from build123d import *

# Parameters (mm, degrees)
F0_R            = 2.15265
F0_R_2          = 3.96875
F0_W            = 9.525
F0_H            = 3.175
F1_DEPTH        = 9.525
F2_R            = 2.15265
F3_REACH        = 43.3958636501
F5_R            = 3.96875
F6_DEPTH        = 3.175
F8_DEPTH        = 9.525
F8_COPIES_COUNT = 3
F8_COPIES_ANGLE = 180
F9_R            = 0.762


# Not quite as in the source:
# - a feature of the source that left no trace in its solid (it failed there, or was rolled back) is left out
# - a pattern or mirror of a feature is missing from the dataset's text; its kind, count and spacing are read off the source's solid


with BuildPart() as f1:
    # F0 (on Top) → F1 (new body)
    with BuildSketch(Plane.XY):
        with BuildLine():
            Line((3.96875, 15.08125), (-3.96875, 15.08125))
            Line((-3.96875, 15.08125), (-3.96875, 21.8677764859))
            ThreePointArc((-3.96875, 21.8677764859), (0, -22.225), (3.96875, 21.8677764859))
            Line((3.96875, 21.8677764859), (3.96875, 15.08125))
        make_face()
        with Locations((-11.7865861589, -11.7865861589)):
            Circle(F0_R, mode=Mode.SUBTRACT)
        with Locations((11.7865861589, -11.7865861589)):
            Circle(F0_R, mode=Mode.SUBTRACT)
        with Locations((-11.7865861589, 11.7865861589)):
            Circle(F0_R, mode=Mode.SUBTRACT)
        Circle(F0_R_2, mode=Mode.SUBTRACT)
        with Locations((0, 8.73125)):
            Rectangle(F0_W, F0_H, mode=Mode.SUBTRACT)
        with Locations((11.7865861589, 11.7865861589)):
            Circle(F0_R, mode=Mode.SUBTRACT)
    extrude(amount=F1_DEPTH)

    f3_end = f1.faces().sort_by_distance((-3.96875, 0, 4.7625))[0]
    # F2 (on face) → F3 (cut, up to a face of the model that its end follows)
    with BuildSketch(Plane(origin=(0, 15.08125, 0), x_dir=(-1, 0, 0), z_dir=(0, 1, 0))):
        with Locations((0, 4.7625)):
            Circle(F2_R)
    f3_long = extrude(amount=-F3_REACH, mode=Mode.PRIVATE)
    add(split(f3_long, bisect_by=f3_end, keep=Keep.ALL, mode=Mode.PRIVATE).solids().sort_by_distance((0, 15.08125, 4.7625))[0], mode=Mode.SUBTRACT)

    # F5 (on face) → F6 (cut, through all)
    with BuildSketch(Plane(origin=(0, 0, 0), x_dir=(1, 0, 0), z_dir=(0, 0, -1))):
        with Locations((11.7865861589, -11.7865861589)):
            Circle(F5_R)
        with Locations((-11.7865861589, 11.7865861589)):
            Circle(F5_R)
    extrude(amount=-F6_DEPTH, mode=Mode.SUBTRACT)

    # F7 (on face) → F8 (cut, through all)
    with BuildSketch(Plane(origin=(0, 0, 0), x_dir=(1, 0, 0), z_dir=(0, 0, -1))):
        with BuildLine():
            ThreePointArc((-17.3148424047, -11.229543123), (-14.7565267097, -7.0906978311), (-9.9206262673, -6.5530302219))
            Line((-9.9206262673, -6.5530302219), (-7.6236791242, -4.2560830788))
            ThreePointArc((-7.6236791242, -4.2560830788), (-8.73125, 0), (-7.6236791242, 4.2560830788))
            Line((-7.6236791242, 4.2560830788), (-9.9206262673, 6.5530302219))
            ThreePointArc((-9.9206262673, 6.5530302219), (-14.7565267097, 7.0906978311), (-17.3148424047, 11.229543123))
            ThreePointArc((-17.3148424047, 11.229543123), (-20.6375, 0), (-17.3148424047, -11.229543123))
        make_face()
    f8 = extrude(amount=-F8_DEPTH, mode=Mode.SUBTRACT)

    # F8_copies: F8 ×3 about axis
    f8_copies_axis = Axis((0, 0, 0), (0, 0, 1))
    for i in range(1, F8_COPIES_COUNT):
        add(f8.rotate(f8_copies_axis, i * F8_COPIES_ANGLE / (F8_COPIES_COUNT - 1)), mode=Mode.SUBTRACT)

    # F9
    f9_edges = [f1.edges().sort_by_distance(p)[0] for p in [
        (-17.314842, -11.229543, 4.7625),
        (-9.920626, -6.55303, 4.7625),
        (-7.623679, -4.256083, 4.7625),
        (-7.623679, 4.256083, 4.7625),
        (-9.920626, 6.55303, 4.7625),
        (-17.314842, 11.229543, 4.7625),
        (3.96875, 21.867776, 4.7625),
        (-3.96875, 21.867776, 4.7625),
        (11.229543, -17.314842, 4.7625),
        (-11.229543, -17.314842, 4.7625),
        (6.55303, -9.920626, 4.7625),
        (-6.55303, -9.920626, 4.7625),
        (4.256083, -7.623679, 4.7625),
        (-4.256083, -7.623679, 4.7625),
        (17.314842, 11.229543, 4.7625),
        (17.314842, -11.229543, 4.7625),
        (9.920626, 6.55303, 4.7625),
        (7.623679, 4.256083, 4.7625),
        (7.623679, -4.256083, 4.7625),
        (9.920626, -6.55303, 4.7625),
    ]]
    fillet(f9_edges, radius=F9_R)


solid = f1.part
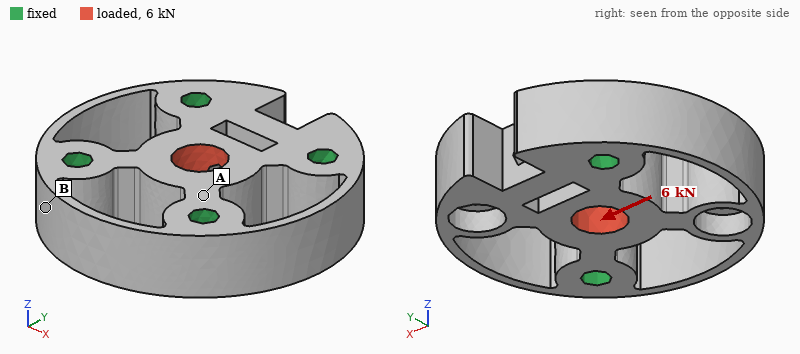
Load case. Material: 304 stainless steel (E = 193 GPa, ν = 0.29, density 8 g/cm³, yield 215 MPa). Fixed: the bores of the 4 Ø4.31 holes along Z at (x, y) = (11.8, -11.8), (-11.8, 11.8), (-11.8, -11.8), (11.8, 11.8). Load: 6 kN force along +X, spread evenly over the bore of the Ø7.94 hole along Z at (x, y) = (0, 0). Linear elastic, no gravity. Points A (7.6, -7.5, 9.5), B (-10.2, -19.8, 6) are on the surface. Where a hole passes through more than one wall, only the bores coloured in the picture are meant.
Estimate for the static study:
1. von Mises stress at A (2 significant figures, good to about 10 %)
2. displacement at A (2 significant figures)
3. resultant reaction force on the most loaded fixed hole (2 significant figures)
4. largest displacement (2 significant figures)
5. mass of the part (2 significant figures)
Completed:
43 MPa
1.3 µm
2.0 kN
4.4 µm
61 g
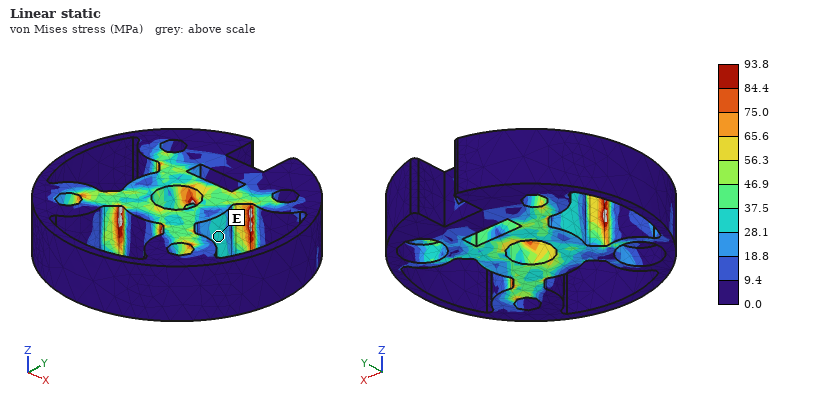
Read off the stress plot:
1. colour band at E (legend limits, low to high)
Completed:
28.1 to 37.5 MPa
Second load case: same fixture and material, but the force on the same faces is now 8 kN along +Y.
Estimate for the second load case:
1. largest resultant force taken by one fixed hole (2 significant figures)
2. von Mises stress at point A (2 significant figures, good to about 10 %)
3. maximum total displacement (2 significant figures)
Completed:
2.4 kN
51 MPa
5.3 µm
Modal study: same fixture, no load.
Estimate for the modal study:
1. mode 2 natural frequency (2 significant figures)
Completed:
28 kHz
